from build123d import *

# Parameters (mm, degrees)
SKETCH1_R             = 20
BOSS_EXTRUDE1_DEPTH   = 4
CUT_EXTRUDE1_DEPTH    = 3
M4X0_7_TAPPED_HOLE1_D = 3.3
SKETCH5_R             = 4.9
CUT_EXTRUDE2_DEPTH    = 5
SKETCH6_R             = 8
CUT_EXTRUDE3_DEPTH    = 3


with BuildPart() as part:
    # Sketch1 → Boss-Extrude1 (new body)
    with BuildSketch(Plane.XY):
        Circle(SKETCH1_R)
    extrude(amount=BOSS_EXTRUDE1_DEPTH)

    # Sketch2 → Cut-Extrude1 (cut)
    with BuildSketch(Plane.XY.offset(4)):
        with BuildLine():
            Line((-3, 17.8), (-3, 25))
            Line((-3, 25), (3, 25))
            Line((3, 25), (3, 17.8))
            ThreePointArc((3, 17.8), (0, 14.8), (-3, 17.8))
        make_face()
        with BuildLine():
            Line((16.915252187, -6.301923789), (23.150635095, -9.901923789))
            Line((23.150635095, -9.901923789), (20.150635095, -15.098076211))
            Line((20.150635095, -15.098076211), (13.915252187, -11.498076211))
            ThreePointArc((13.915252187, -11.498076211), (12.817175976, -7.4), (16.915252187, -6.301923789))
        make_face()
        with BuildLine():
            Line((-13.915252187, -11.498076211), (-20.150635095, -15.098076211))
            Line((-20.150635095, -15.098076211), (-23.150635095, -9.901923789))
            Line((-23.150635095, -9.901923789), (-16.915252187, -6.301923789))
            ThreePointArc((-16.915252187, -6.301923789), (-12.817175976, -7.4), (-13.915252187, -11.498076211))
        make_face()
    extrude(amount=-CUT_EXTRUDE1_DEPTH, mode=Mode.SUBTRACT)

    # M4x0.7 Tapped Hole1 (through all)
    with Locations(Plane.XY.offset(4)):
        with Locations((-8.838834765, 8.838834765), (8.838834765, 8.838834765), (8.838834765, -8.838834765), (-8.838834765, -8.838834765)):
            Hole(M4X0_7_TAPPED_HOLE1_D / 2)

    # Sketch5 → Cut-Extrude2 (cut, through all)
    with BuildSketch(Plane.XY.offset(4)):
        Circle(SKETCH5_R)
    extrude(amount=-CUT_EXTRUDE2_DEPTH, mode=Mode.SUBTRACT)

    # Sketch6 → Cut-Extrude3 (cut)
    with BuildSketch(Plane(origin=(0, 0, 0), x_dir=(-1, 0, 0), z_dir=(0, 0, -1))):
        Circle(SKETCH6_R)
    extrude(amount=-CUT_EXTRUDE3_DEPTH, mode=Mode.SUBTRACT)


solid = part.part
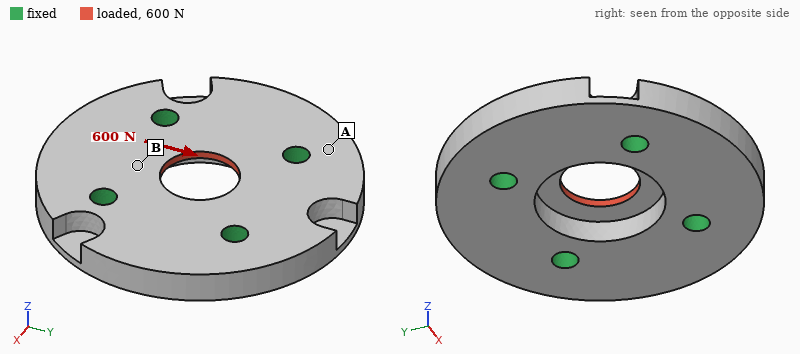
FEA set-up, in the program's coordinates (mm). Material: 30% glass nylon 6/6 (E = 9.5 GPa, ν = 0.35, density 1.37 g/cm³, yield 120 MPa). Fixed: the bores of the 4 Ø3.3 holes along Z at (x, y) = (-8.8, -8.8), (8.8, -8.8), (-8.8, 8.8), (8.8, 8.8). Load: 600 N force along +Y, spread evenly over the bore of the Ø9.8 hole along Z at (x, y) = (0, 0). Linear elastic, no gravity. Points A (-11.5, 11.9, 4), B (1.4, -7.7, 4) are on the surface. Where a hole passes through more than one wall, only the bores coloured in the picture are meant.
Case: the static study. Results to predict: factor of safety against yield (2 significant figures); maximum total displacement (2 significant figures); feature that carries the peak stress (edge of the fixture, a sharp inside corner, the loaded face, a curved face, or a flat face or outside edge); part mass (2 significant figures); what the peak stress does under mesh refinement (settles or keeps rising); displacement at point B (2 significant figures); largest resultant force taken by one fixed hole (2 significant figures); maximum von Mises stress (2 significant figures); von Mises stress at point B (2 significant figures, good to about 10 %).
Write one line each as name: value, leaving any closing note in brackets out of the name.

factor of safety against yield: 3.5
maximum total displacement: 20 µm
feature that carries the peak stress: the loaded face
part mass: 5.4 g
what the peak stress does under mesh refinement: settles
displacement at point B: 11 µm
largest resultant force taken by one fixed hole: 150 N
maximum von Mises stress: 34 MPa
von Mises stress at point B: 15 MPa
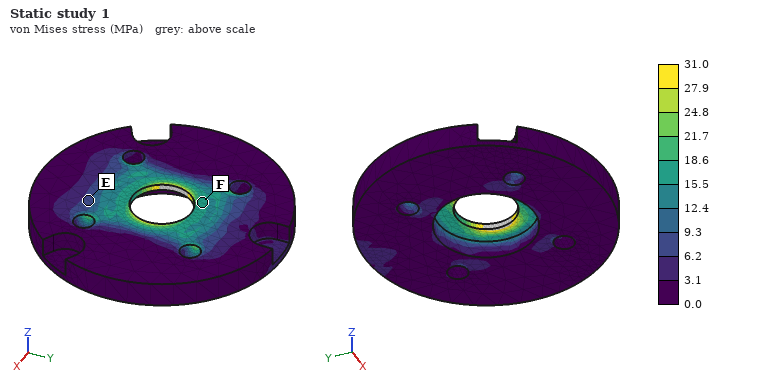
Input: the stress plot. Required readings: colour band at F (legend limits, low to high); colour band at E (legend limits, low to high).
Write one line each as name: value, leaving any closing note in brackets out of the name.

colour band at F: 15.5 to 18.6 MPa
colour band at E: 6.2 to 9.3 MPa
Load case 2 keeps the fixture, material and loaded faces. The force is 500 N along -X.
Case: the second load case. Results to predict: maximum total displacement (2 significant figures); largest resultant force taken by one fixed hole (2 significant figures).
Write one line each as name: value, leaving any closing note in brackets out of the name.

maximum total displacement: 17 µm
largest resultant force taken by one fixed hole: 130 N
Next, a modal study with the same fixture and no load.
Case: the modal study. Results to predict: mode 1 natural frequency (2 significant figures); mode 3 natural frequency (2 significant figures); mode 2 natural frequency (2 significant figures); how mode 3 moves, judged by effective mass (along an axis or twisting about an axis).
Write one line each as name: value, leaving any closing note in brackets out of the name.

mode 1 natural frequency: 13 kHz
mode 3 natural frequency: 14 kHz
mode 2 natural frequency: 13 kHz
how mode 3 moves, judged by effective mass: along Z
